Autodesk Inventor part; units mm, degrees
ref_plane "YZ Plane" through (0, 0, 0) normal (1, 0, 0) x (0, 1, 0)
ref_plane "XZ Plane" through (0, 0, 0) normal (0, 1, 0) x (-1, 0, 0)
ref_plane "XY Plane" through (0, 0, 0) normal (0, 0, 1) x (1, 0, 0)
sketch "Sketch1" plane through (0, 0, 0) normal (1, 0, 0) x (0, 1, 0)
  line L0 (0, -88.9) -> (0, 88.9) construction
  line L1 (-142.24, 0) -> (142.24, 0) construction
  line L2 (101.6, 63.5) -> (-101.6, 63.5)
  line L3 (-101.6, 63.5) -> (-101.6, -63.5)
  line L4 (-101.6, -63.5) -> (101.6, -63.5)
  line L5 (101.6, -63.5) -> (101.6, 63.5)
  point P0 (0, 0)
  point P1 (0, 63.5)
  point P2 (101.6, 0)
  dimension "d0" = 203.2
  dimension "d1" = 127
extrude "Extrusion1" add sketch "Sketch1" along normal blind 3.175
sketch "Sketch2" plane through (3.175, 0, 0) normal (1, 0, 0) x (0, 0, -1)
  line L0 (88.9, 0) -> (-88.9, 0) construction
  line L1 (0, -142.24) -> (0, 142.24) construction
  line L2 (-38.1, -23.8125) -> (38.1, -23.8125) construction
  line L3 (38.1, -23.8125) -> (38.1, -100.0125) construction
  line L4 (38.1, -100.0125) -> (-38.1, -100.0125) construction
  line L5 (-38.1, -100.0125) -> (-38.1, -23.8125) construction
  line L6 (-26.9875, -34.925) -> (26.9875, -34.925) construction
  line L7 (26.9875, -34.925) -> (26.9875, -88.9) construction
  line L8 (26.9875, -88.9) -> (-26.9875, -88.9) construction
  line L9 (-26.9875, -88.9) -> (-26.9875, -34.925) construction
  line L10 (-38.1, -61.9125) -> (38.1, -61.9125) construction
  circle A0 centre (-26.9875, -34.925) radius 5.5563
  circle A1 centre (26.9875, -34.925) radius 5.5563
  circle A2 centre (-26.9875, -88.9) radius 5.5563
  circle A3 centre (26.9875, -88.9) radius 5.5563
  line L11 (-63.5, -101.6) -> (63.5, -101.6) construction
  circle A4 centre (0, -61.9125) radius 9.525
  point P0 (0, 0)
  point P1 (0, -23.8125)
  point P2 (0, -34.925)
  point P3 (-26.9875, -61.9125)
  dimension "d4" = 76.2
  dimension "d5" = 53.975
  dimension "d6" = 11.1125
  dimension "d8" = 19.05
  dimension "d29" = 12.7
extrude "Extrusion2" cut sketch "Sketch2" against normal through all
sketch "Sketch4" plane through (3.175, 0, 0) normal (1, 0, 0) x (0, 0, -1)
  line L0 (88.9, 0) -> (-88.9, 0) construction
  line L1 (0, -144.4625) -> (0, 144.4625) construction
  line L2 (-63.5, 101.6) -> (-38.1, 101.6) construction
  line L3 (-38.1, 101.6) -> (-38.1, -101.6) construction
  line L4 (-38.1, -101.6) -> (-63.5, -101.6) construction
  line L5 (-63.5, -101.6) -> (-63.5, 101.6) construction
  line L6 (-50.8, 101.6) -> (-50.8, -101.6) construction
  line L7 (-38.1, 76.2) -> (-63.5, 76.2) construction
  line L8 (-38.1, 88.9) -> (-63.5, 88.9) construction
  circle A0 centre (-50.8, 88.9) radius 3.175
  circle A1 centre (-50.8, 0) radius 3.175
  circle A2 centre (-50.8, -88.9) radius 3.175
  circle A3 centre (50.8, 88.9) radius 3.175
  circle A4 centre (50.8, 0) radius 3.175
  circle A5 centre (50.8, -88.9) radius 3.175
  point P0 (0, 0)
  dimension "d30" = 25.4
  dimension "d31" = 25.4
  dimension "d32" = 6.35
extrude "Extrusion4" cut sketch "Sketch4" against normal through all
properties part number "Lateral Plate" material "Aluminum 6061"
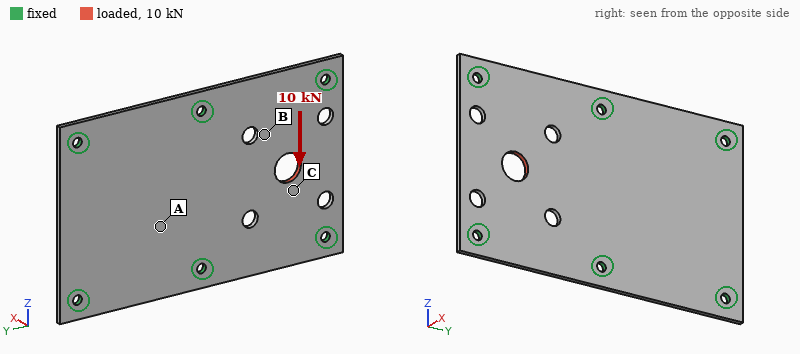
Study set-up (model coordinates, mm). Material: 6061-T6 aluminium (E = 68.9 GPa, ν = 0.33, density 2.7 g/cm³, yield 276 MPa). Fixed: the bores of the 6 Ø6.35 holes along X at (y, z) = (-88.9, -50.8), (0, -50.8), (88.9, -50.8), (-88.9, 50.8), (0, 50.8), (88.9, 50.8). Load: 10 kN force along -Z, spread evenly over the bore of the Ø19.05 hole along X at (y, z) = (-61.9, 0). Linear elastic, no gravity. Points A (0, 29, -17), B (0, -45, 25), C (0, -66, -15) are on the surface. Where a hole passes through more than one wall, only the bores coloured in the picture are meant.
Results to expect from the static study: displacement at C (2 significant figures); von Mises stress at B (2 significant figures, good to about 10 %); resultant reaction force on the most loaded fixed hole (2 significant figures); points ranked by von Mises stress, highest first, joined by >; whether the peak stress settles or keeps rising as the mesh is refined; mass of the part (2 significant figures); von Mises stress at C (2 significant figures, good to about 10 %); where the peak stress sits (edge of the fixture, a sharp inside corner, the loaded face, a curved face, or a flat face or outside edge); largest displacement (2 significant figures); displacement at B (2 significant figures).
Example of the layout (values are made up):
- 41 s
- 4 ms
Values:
- 31 µm
- 29 MPa
- 3.3 kN
- C > B > A
- keeps rising
- 210 g
- 49 MPa
- edge of the fixture
- 39 µm
- 26 µm
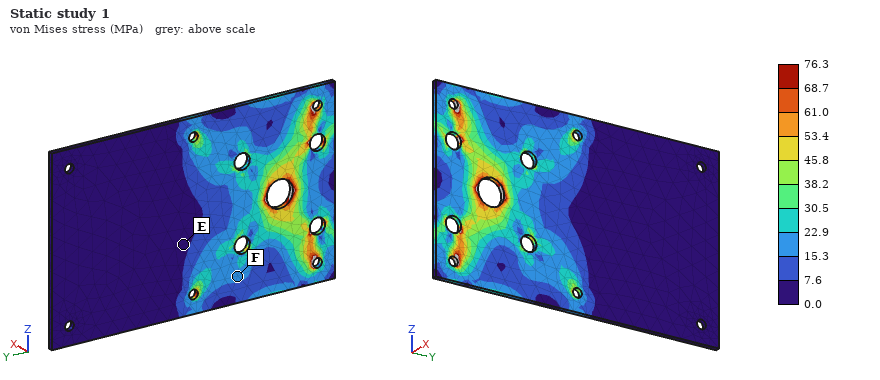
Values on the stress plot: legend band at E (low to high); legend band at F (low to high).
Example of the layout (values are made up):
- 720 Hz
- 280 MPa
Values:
- 0.0 to 7.6 MPa
- 15.3 to 22.9 MPa
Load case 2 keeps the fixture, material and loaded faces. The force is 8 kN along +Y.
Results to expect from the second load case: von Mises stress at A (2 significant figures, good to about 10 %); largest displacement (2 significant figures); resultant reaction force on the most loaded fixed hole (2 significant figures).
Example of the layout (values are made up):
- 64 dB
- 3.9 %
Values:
- 7.1 MPa
- 42 µm
- 1.9 kN
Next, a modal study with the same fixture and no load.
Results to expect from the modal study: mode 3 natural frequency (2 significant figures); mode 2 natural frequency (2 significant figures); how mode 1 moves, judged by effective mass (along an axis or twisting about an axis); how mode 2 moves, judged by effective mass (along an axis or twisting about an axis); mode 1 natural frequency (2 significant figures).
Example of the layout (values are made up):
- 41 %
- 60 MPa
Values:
- 2000 Hz
- 1300 Hz
- along X
- twisting about Z
- 1200 Hz
